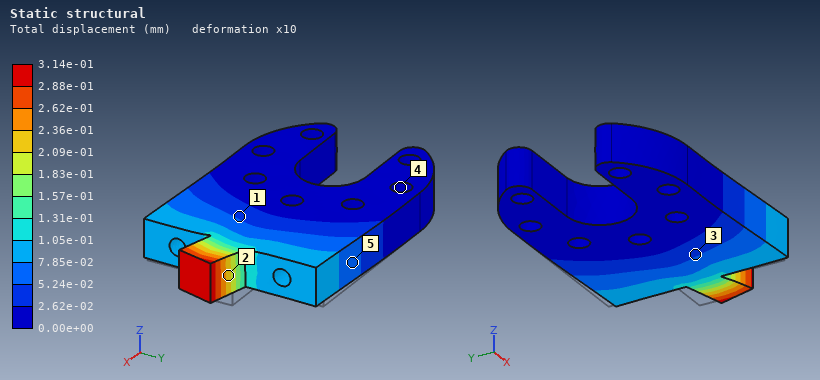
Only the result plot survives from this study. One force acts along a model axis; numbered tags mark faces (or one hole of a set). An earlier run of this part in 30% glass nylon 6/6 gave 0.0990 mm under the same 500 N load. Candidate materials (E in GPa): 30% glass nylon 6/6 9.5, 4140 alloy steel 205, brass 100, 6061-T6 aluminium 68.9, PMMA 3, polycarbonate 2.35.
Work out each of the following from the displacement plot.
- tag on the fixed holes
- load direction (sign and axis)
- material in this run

4
-Y
PMMA
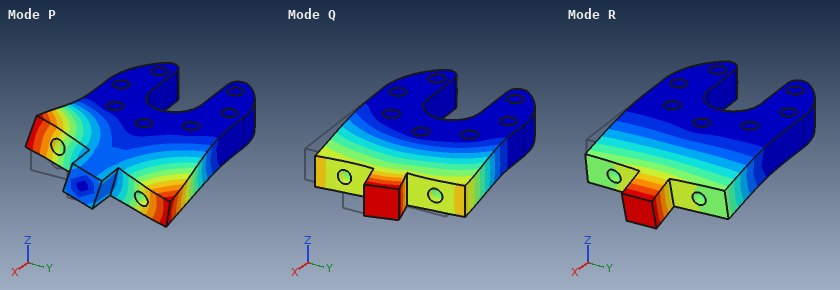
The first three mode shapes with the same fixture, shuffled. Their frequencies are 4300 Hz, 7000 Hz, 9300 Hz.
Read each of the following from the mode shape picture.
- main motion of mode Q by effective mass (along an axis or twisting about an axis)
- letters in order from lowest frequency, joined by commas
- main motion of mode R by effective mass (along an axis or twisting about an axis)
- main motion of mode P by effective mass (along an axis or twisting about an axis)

along Y
R, P, Q
along Z
twisting about X
